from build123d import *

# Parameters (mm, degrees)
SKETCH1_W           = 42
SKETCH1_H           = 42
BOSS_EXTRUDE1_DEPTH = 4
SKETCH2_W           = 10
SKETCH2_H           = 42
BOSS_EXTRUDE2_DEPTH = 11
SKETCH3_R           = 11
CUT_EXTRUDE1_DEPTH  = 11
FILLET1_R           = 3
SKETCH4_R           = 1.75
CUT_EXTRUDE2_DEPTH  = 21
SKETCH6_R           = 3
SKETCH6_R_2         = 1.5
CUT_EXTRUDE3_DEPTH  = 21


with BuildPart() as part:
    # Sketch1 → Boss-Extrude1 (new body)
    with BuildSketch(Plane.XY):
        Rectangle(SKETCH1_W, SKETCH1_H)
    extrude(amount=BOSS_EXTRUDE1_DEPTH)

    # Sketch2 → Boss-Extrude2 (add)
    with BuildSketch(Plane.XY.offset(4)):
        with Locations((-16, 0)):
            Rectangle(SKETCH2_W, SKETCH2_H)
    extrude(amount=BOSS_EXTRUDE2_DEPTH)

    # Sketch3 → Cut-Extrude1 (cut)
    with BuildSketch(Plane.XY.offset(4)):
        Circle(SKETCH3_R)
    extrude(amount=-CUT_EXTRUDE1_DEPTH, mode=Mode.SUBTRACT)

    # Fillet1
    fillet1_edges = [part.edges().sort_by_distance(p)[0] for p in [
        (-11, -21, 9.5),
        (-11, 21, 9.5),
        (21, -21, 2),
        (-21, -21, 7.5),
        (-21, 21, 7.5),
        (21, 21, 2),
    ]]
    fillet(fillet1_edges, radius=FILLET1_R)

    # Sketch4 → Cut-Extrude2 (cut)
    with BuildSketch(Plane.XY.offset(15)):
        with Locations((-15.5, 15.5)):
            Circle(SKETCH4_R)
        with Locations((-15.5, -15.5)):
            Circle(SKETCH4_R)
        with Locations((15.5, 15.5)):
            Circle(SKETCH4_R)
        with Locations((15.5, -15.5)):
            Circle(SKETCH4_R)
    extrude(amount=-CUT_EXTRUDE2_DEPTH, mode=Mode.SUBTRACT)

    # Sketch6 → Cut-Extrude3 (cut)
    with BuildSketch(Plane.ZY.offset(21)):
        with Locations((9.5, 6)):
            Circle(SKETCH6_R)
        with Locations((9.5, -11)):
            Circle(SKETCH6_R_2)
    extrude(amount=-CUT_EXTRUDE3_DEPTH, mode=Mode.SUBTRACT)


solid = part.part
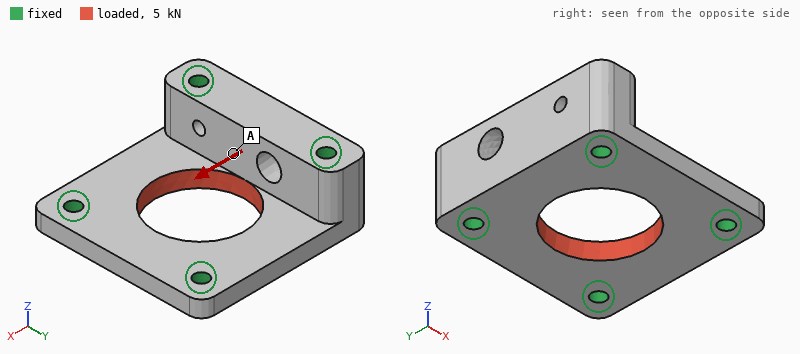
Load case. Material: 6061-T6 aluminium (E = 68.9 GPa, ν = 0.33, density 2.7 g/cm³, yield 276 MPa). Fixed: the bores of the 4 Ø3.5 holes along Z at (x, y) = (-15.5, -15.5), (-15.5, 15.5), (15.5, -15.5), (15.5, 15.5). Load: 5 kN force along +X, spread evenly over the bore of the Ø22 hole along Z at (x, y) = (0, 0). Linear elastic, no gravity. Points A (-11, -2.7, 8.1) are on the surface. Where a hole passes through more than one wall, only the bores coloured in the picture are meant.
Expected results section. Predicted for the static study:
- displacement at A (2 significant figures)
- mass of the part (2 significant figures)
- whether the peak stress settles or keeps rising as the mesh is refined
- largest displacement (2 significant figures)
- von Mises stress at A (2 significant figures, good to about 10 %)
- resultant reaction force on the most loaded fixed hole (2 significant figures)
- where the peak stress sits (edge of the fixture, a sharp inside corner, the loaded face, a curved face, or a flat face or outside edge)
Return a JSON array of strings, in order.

["3.8 µm", "25 g", "keeps rising", "12 µm", "9.7 MPa", "1.4 kN", "edge of the fixture"]
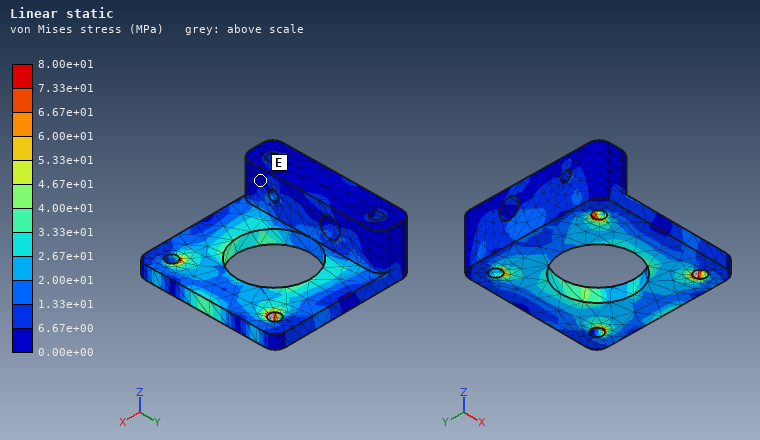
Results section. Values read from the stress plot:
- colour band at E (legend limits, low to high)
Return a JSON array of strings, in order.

["0.00e+00 to 6.67e+00 MPa"]
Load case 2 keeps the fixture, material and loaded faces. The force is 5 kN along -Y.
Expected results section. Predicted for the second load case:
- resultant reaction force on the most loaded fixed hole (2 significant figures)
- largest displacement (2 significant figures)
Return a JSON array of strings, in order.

["1.4 kN", "10 µm"]
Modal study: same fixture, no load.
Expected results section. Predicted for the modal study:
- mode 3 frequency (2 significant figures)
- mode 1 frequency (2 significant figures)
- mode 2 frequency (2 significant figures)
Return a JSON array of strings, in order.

["25 kHz", "21 kHz", "24 kHz"]
